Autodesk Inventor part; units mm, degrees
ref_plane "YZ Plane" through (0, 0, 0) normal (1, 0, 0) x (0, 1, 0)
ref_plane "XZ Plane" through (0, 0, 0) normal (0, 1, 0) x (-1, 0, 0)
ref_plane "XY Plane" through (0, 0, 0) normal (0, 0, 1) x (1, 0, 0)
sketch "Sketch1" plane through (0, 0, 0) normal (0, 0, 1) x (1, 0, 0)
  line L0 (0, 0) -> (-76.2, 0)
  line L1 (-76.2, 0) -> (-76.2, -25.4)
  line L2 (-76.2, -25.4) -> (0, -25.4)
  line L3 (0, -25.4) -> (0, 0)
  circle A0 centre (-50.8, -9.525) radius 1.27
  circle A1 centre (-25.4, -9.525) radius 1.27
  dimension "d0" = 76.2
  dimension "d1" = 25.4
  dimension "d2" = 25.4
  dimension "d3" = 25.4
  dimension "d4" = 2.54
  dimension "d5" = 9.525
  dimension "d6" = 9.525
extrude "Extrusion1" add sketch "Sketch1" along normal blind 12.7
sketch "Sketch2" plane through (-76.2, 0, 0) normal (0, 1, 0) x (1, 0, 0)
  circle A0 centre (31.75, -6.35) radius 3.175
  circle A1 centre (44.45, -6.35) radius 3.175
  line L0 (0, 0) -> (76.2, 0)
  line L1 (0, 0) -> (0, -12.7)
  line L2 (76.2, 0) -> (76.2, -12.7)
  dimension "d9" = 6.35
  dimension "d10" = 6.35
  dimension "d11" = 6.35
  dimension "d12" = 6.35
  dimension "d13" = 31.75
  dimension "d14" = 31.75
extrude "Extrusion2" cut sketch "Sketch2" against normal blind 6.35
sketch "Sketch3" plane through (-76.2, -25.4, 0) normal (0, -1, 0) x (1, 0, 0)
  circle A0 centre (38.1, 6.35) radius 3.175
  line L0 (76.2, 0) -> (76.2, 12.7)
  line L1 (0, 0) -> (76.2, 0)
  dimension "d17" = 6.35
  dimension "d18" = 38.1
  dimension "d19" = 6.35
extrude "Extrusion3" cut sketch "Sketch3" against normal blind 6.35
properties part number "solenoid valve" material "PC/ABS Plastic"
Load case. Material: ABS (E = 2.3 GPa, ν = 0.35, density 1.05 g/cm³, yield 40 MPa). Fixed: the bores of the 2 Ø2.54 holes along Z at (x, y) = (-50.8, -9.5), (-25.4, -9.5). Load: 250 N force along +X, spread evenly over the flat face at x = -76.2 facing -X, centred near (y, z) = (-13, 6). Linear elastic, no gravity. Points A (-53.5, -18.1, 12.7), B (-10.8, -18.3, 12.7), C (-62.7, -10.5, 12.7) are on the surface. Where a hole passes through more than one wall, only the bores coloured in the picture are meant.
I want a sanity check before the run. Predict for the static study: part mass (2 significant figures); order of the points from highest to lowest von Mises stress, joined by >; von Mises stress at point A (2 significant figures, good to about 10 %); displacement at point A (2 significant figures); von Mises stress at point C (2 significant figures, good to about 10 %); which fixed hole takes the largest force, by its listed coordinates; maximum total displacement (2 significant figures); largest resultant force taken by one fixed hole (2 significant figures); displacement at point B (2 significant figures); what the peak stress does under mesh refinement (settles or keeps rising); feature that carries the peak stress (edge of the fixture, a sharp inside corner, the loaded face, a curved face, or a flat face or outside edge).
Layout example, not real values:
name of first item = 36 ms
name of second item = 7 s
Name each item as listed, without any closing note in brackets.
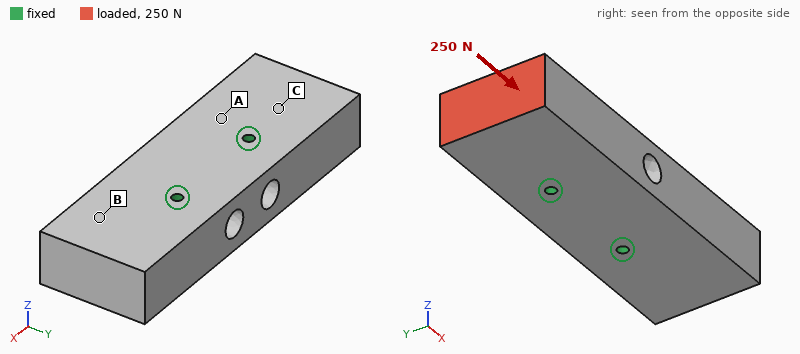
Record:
part mass = 25 g
order of the points from highest to lowest von Mises stress, joined by > = C > A > B
von Mises stress at point A = 0.60 MPa
displacement at point A = 6.6 µm
von Mises stress at point C = 0.95 MPa
which fixed hole takes the largest force, by its listed coordinates = (-50.8, -9.5)
maximum total displacement = 18 µm
largest resultant force taken by one fixed hole = 190 N
displacement at point B = 2.9 µm
what the peak stress does under mesh refinement = keeps rising
feature that carries the peak stress = edge of the fixture
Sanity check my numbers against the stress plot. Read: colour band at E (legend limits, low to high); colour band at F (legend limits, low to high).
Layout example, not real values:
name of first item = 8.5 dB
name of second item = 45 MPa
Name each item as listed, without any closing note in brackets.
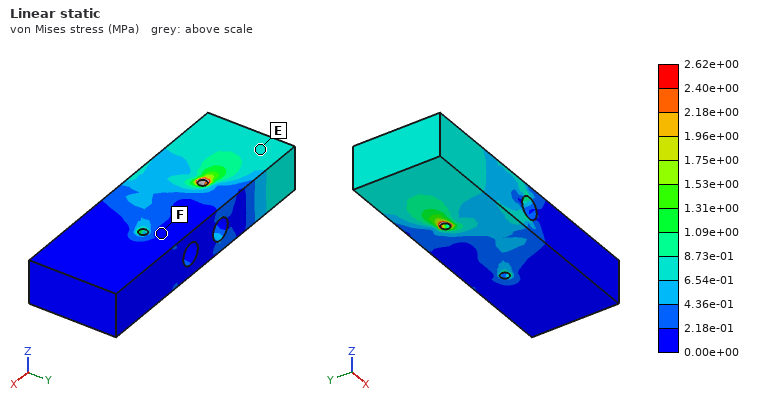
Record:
colour band at E = 6.54e-01 to 8.73e-01 MPa
colour band at F = 0.00e+00 to 2.18e-01 MPa
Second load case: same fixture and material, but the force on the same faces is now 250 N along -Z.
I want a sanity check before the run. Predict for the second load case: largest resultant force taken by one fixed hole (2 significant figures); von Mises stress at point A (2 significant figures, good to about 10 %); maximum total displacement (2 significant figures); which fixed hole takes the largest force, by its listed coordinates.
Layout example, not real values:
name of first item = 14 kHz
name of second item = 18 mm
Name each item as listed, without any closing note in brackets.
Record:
largest resultant force taken by one fixed hole = 350 N
von Mises stress at point A = 5.8 MPa
maximum total displacement = 0.26 mm
which fixed hole takes the largest force, by its listed coordinates = (-50.8, -9.5)
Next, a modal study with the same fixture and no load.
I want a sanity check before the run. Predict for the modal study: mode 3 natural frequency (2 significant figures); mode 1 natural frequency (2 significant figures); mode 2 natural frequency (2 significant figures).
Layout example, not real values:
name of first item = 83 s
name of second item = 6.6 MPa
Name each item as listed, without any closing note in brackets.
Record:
mode 3 natural frequency = 3500 Hz
mode 1 natural frequency = 3100 Hz
mode 2 natural frequency = 3200 Hz
